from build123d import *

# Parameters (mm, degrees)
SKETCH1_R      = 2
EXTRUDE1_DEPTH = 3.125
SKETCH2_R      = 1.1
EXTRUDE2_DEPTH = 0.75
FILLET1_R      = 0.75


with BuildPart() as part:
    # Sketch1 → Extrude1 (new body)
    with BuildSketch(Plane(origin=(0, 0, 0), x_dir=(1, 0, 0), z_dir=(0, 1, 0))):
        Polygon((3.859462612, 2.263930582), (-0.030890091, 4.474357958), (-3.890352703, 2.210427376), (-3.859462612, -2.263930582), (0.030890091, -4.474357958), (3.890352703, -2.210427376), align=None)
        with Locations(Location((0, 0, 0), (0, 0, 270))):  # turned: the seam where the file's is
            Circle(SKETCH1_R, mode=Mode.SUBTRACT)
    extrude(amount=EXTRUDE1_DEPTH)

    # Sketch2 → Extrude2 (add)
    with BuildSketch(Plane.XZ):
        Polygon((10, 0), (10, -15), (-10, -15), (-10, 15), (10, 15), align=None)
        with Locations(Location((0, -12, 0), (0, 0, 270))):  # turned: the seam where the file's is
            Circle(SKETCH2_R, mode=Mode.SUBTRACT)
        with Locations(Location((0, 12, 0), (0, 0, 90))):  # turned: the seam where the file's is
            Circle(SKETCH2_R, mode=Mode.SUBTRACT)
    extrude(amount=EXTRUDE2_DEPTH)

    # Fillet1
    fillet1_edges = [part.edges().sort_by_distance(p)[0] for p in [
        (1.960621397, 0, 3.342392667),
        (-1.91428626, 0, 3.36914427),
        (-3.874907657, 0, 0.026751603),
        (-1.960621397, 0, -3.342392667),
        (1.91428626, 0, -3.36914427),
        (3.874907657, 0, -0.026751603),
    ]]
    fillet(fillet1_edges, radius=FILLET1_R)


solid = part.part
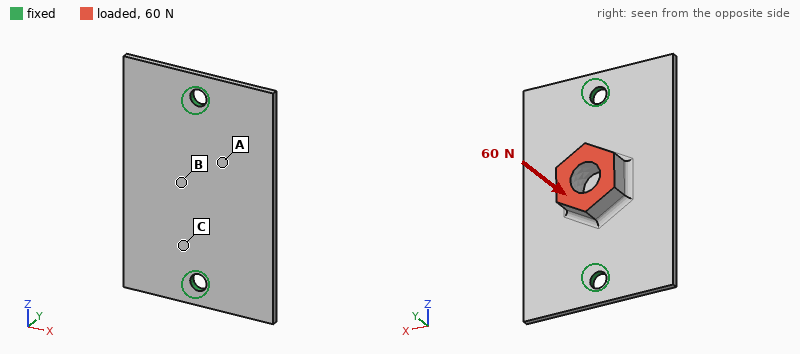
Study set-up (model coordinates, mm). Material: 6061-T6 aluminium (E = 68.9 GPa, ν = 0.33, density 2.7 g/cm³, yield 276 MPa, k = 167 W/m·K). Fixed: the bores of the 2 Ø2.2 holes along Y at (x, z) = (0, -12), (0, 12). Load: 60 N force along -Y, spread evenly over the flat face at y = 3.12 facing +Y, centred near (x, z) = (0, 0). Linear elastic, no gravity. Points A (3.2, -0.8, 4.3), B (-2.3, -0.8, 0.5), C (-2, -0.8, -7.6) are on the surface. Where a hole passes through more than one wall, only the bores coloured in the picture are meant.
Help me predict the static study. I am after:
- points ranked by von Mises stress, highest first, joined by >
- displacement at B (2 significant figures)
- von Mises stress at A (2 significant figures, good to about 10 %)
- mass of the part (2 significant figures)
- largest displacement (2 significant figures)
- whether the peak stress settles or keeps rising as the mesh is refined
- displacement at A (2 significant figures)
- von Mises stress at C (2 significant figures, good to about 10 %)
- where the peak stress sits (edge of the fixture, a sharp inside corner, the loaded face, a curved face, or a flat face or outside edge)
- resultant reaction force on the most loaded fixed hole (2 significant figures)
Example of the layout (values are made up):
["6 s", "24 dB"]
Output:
["A > C > B", "47 µm", "48 MPa", "1.5 g", "51 µm", "keeps rising", "44 µm", "27 MPa", "edge of the fixture", "35 N"]
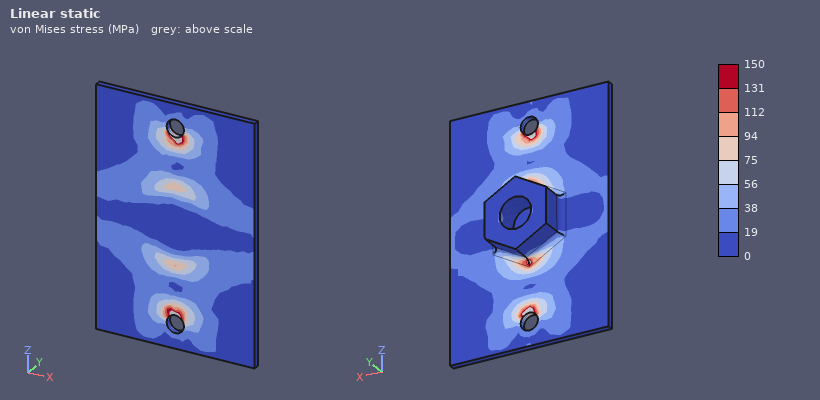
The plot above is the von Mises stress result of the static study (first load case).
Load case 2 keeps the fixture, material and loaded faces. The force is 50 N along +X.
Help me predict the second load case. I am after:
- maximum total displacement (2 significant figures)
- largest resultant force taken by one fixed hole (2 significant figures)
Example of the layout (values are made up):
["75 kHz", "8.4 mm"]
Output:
["95 µm", "25 N"]
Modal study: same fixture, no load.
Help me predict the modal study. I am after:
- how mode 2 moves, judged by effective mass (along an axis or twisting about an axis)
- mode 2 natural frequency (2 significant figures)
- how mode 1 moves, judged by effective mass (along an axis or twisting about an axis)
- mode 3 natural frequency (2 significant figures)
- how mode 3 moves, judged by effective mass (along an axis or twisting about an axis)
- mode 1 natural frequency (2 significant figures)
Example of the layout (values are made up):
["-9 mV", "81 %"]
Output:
["along Y", "5700 Hz", "twisting about Z", "8900 Hz", "twisting about X", "4100 Hz"]
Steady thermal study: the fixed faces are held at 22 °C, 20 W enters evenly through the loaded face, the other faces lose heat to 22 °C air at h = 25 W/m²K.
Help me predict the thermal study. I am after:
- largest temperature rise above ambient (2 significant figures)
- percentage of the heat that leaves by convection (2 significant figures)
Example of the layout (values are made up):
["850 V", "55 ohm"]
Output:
["64 K", "5.5 %"]
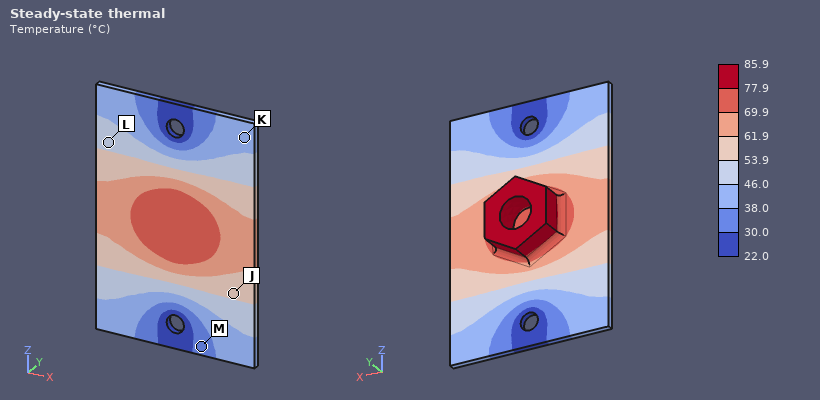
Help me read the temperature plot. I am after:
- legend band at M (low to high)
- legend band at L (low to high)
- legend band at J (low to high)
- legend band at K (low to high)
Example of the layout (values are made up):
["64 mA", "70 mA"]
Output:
["30.0 to 38.0 °C", "46.0 to 53.9 °C", "53.9 to 61.9 °C", "38.0 to 46.0 °C"]
